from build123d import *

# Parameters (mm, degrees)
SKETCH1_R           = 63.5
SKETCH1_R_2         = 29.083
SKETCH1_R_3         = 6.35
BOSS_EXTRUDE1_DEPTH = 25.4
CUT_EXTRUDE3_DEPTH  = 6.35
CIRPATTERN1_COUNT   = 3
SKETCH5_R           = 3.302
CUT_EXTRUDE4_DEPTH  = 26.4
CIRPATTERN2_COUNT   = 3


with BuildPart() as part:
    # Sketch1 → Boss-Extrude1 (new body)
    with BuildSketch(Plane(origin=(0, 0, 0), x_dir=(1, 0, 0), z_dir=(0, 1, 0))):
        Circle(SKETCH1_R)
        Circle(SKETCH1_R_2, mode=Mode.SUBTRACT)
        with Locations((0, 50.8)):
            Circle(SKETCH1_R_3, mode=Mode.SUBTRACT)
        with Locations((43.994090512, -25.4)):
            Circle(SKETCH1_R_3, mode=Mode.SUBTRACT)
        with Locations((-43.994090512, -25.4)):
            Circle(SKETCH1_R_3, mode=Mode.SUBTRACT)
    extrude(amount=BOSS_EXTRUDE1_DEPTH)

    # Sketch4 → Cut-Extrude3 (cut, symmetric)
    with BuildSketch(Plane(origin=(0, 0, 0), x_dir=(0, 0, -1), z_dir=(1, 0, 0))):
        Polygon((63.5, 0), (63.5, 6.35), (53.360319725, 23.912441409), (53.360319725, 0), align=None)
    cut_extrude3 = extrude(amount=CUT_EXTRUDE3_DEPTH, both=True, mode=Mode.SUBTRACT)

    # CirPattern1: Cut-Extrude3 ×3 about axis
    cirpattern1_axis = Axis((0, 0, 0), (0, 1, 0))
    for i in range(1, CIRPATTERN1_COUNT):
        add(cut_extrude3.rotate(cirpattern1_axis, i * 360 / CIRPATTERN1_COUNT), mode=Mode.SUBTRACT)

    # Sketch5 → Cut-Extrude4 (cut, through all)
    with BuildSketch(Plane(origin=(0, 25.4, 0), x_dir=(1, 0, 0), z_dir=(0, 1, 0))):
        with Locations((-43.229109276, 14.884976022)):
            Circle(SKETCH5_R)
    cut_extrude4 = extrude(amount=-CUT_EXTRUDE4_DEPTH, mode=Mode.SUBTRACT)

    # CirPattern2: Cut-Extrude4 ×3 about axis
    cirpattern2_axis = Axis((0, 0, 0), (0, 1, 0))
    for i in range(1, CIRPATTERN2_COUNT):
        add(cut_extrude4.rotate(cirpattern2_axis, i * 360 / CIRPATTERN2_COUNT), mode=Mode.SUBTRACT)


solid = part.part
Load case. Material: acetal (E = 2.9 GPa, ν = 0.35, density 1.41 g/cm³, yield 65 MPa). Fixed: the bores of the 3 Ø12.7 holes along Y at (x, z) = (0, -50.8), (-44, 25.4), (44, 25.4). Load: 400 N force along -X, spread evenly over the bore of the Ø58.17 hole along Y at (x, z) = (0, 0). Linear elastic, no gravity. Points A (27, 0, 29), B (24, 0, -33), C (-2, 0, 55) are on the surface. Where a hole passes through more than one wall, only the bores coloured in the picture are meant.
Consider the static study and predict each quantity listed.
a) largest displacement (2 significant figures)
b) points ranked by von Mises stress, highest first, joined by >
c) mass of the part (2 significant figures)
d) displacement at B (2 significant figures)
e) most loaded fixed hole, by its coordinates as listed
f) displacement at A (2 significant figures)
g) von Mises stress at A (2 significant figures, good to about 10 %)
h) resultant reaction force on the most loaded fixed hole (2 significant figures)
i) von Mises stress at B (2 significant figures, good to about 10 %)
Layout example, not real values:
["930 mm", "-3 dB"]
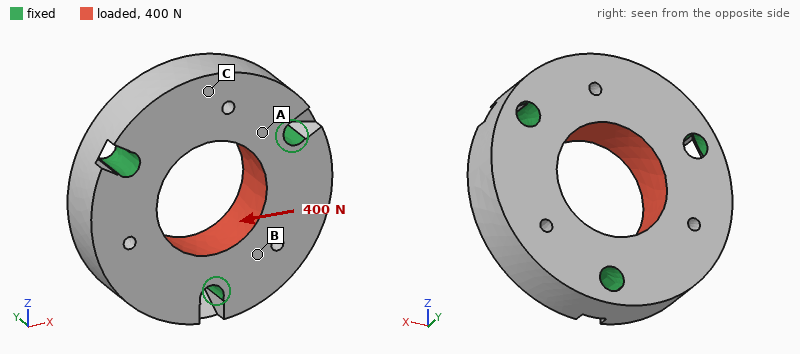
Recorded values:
["3.1 µm", "A > B > C", "340 g", "2.1 µm", "(0, -50.8)", "0.61 µm", "0.16 MPa", "160 N", "0.098 MPa"]
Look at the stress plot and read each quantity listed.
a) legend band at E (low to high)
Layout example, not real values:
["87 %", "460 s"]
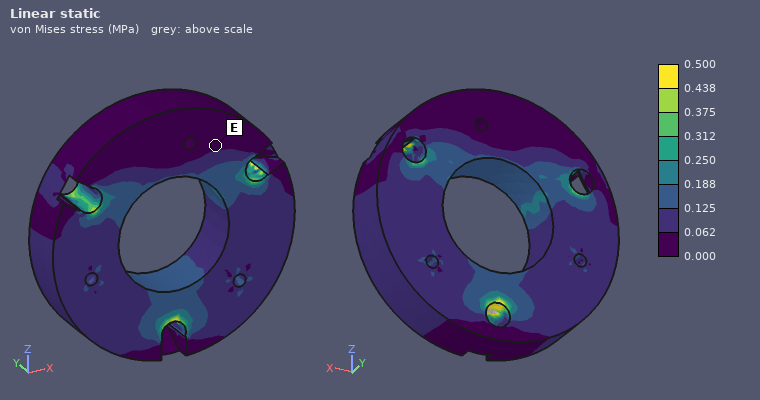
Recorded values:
["0.000 to 0.062 MPa"]
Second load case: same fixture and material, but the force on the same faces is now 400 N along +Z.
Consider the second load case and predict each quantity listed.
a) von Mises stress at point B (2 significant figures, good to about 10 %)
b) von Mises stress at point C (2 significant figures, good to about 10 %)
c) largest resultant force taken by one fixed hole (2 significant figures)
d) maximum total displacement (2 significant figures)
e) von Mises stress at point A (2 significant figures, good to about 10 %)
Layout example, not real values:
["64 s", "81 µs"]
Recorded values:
["0.073 MPa", "0.12 MPa", "150 N", "3.4 µm", "0.11 MPa"]
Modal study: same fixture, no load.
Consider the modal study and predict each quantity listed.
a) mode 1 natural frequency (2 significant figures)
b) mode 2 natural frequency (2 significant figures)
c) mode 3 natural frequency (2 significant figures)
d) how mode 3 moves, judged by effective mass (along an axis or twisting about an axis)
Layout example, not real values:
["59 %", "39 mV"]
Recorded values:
["2400 Hz", "2400 Hz", "2600 Hz", "along Y"]
